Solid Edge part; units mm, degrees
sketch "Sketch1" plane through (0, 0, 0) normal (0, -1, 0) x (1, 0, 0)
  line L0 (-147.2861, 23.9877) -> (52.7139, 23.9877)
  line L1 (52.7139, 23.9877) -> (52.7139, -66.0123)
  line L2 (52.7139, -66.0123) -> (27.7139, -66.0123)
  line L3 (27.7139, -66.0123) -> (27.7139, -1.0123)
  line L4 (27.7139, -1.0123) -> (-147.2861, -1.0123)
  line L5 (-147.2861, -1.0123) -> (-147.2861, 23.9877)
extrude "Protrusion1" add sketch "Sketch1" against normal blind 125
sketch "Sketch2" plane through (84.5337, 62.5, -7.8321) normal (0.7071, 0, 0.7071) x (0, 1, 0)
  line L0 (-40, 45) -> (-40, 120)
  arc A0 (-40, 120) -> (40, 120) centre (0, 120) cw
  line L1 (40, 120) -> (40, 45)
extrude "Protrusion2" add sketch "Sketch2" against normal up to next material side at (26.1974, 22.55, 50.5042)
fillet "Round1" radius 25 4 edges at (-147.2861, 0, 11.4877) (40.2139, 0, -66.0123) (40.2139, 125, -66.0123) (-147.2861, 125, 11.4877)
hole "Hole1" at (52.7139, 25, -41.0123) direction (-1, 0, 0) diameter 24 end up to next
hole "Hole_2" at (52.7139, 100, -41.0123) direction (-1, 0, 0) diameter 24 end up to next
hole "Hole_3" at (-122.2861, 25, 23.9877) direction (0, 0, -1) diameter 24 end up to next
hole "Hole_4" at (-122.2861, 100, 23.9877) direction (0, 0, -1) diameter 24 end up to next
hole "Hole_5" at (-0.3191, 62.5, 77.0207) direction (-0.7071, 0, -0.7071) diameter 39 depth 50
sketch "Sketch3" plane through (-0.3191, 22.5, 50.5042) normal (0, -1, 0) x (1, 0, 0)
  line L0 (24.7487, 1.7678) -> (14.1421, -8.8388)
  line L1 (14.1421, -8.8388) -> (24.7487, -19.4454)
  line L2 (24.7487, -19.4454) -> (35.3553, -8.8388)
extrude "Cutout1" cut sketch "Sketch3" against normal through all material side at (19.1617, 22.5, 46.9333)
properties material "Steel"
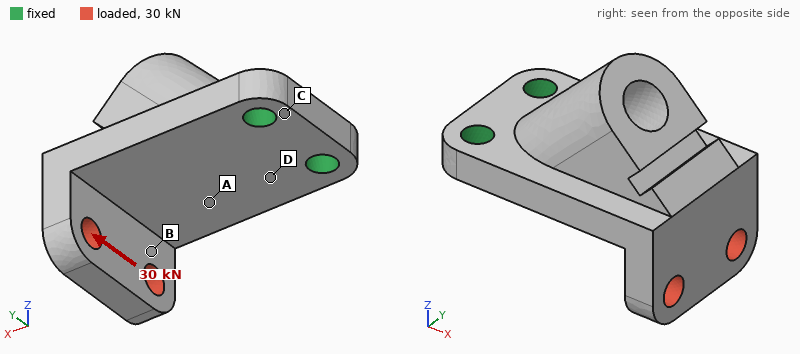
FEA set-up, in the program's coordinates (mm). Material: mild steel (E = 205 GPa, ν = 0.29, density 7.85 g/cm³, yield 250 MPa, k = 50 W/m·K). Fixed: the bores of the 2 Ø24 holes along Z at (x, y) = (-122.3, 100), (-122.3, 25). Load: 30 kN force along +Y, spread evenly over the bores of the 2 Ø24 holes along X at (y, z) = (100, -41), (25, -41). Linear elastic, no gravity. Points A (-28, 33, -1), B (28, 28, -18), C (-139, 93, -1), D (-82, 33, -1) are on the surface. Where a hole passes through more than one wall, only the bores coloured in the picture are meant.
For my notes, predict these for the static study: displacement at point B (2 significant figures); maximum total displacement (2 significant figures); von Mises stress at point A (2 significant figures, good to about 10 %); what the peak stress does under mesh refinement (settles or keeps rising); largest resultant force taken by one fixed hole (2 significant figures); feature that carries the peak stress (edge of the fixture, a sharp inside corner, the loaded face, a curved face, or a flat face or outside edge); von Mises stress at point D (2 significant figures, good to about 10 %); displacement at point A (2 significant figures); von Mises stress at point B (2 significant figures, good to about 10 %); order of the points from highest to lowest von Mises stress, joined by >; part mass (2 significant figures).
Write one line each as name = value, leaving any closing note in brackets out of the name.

displacement at point B = 0.13 mm
maximum total displacement = 0.22 mm
von Mises stress at point A = 58 MPa
what the peak stress does under mesh refinement = keeps rising
largest resultant force taken by one fixed hole = 59 kN
feature that carries the peak stress = edge of the fixture
von Mises stress at point D = 75 MPa
displacement at point A = 0.056 mm
von Mises stress at point B = 44 MPa
order of the points from highest to lowest von Mises stress, joined by > = D > A > B > C
part mass = 9.0 kg
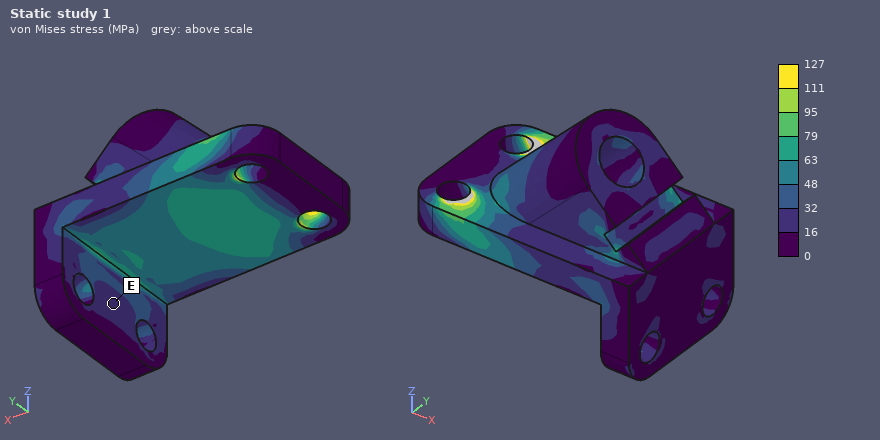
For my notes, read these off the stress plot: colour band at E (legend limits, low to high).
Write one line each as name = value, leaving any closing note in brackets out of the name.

colour band at E = 16 to 32 MPa
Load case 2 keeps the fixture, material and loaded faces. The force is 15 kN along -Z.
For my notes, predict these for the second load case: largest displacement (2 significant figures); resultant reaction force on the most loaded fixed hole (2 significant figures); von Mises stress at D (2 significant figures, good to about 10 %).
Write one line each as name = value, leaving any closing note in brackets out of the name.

largest displacement = 0.41 mm
resultant reaction force on the most loaded fixed hole = 8.0 kN
von Mises stress at D = 79 MPa
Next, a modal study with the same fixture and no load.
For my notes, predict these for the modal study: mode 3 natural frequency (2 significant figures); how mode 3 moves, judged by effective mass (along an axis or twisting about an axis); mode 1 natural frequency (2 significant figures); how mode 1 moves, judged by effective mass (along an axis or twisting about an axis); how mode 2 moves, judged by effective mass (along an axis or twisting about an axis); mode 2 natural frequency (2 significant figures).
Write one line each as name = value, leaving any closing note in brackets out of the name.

mode 3 natural frequency = 2000 Hz
how mode 3 moves, judged by effective mass = along Y
mode 1 natural frequency = 530 Hz
how mode 1 moves, judged by effective mass = along Z
how mode 2 moves, judged by effective mass = along Y
mode 2 natural frequency = 1500 Hz
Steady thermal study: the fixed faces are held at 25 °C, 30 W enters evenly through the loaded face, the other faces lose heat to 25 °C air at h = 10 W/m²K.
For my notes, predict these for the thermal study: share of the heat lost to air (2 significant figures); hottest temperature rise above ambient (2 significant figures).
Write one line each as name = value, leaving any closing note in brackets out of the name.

share of the heat lost to air = 35 %
hottest temperature rise above ambient = 26 K
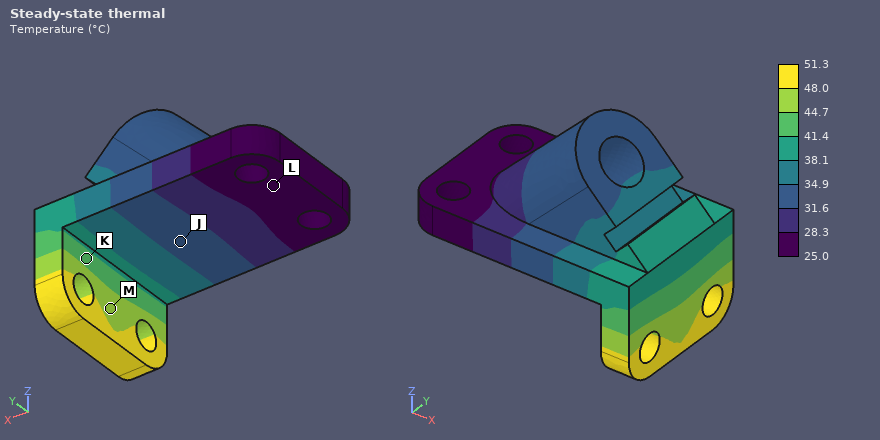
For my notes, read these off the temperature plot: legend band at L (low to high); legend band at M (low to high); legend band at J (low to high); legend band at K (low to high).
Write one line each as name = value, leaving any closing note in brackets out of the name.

legend band at L = 25.0 to 28.3 °C
legend band at M = 44.7 to 48.0 °C
legend band at J = 31.6 to 34.9 °C
legend band at K = 41.4 to 44.7 °C
